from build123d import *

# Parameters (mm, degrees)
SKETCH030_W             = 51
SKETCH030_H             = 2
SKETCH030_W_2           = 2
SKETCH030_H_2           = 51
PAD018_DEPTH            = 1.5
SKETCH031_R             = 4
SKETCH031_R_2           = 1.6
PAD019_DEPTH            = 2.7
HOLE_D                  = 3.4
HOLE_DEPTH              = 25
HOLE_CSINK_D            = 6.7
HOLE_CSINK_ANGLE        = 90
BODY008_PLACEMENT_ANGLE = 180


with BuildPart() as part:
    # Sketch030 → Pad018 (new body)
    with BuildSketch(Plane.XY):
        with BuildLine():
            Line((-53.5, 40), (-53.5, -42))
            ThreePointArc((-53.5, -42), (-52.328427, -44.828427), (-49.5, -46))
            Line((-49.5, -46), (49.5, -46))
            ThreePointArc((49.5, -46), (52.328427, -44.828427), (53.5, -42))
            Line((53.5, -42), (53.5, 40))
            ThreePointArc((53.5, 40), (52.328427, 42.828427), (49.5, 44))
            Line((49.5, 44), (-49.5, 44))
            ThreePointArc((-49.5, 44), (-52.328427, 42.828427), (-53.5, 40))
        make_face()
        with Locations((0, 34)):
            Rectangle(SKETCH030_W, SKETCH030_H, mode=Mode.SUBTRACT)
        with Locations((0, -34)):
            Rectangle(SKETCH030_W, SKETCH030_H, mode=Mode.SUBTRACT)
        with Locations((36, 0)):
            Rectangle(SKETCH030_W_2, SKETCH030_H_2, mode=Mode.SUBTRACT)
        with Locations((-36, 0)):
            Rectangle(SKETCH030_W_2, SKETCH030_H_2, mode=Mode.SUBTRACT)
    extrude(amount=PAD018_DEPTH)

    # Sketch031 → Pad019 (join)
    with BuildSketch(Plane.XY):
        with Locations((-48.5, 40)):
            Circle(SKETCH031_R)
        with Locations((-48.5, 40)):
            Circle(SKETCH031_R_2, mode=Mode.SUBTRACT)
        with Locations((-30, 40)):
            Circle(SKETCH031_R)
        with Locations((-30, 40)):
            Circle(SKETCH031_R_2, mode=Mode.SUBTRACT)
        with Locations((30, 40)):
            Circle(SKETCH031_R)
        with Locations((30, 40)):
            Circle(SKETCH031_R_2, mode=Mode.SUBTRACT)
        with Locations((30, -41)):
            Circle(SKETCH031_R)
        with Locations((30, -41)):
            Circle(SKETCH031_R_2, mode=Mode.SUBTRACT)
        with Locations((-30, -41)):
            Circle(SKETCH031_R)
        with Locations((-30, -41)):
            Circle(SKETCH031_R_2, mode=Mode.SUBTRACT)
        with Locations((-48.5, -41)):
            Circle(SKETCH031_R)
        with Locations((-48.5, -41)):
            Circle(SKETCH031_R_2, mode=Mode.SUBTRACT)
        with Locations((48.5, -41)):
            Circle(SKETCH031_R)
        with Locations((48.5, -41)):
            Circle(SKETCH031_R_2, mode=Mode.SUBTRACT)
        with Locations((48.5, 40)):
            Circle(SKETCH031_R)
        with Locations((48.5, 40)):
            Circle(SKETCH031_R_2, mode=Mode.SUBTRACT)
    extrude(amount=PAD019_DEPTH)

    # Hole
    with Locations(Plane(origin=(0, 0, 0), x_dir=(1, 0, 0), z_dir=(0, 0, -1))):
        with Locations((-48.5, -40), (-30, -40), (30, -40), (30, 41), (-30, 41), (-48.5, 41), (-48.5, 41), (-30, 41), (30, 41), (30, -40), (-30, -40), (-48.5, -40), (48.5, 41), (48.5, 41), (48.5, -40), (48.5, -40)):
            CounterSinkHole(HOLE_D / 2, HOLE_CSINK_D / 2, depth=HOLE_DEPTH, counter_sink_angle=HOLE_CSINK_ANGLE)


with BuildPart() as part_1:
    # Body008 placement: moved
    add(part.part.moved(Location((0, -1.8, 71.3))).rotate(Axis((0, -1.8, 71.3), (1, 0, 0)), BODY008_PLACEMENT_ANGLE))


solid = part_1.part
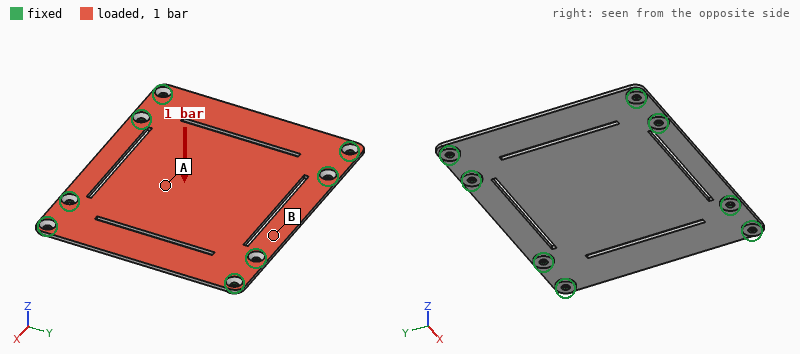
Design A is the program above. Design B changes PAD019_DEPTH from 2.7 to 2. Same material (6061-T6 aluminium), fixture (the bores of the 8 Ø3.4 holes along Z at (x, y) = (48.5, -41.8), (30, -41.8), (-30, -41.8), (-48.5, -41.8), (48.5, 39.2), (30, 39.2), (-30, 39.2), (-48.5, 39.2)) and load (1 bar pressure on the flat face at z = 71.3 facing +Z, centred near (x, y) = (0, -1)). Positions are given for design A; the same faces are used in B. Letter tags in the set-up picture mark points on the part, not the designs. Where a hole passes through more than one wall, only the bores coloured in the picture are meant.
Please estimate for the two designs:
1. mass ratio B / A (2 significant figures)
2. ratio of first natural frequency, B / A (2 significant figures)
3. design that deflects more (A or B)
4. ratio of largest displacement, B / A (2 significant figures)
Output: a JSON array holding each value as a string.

["0.98", "0.94", "B", "1.1"]
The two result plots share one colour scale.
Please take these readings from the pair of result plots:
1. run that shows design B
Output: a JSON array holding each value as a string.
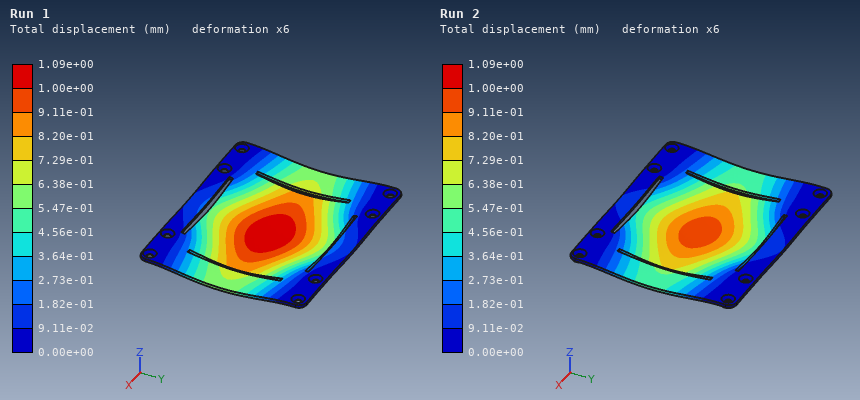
["Run 1"]
